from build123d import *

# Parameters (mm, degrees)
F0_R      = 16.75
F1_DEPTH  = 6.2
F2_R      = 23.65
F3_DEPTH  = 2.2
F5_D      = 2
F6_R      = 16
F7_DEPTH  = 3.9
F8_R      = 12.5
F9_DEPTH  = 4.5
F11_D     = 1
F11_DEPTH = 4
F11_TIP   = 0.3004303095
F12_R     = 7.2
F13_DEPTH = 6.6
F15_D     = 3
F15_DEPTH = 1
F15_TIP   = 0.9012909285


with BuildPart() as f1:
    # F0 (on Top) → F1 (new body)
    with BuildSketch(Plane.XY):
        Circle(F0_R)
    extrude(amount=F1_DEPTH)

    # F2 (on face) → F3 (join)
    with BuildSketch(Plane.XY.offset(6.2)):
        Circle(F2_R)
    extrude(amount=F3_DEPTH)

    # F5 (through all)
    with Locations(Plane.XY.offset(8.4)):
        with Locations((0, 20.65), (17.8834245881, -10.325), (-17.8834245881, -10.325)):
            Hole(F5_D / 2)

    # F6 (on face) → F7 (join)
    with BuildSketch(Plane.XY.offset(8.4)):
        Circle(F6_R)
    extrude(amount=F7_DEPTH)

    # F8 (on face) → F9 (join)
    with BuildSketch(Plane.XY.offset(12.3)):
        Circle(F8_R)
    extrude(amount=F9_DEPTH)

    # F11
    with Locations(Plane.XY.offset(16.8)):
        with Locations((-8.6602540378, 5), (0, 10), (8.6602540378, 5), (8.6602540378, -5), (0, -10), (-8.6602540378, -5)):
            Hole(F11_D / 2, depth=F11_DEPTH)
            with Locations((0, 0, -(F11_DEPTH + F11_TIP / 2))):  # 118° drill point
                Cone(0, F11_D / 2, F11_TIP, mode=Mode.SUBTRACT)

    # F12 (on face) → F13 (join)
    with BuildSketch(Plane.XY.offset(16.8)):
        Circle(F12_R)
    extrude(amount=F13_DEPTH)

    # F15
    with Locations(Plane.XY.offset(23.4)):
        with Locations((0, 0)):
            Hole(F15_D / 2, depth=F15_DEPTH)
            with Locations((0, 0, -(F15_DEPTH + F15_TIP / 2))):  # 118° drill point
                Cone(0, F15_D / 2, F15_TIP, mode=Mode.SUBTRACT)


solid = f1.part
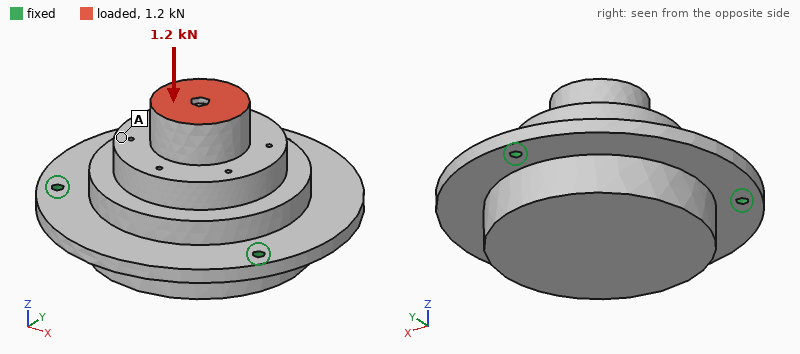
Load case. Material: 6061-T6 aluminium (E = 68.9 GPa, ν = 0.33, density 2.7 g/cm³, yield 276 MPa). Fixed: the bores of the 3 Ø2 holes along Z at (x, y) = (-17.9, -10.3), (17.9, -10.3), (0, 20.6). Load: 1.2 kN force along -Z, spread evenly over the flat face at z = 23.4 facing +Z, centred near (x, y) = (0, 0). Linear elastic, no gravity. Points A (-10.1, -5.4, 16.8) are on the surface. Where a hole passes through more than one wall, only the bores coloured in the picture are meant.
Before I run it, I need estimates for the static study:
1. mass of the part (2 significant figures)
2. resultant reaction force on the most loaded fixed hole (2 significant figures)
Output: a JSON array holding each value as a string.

["42 g", "400 N"]
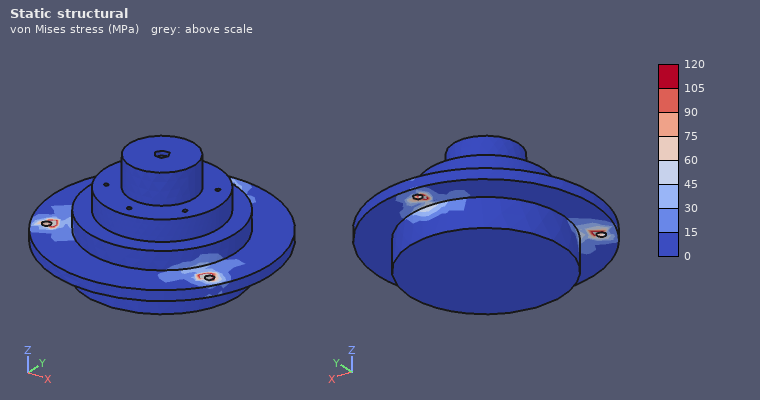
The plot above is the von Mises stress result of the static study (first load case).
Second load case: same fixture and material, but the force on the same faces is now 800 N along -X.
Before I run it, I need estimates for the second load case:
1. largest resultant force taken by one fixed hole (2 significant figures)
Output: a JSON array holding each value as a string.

["480 N"]
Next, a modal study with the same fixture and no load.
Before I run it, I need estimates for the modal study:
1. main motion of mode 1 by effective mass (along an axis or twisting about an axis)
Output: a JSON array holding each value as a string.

["along Z"]
